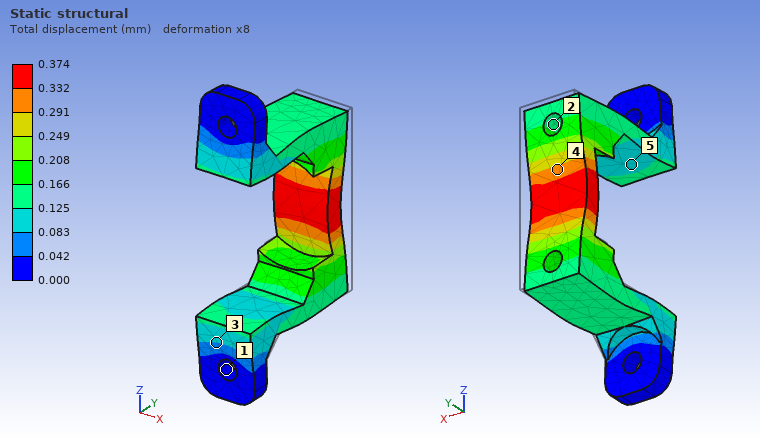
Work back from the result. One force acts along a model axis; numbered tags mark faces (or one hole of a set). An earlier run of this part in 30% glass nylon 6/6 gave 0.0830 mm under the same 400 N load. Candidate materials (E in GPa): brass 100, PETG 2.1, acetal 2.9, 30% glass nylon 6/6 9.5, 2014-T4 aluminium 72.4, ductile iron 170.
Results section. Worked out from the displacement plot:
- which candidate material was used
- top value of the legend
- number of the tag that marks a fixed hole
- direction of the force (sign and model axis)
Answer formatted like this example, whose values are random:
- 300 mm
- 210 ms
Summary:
- PETG
- 0.374 mm
- 1
- -Y
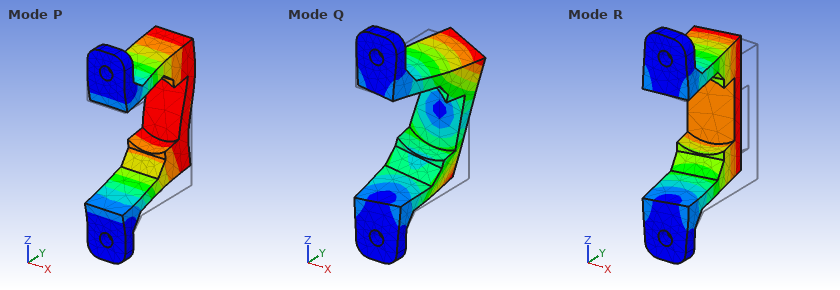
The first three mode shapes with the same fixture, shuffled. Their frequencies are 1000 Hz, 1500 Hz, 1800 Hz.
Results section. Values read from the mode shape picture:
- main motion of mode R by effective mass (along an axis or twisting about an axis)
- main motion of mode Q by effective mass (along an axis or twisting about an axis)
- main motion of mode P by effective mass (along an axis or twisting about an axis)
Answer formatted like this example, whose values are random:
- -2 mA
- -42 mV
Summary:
- along X
- twisting about Y
- along Z
